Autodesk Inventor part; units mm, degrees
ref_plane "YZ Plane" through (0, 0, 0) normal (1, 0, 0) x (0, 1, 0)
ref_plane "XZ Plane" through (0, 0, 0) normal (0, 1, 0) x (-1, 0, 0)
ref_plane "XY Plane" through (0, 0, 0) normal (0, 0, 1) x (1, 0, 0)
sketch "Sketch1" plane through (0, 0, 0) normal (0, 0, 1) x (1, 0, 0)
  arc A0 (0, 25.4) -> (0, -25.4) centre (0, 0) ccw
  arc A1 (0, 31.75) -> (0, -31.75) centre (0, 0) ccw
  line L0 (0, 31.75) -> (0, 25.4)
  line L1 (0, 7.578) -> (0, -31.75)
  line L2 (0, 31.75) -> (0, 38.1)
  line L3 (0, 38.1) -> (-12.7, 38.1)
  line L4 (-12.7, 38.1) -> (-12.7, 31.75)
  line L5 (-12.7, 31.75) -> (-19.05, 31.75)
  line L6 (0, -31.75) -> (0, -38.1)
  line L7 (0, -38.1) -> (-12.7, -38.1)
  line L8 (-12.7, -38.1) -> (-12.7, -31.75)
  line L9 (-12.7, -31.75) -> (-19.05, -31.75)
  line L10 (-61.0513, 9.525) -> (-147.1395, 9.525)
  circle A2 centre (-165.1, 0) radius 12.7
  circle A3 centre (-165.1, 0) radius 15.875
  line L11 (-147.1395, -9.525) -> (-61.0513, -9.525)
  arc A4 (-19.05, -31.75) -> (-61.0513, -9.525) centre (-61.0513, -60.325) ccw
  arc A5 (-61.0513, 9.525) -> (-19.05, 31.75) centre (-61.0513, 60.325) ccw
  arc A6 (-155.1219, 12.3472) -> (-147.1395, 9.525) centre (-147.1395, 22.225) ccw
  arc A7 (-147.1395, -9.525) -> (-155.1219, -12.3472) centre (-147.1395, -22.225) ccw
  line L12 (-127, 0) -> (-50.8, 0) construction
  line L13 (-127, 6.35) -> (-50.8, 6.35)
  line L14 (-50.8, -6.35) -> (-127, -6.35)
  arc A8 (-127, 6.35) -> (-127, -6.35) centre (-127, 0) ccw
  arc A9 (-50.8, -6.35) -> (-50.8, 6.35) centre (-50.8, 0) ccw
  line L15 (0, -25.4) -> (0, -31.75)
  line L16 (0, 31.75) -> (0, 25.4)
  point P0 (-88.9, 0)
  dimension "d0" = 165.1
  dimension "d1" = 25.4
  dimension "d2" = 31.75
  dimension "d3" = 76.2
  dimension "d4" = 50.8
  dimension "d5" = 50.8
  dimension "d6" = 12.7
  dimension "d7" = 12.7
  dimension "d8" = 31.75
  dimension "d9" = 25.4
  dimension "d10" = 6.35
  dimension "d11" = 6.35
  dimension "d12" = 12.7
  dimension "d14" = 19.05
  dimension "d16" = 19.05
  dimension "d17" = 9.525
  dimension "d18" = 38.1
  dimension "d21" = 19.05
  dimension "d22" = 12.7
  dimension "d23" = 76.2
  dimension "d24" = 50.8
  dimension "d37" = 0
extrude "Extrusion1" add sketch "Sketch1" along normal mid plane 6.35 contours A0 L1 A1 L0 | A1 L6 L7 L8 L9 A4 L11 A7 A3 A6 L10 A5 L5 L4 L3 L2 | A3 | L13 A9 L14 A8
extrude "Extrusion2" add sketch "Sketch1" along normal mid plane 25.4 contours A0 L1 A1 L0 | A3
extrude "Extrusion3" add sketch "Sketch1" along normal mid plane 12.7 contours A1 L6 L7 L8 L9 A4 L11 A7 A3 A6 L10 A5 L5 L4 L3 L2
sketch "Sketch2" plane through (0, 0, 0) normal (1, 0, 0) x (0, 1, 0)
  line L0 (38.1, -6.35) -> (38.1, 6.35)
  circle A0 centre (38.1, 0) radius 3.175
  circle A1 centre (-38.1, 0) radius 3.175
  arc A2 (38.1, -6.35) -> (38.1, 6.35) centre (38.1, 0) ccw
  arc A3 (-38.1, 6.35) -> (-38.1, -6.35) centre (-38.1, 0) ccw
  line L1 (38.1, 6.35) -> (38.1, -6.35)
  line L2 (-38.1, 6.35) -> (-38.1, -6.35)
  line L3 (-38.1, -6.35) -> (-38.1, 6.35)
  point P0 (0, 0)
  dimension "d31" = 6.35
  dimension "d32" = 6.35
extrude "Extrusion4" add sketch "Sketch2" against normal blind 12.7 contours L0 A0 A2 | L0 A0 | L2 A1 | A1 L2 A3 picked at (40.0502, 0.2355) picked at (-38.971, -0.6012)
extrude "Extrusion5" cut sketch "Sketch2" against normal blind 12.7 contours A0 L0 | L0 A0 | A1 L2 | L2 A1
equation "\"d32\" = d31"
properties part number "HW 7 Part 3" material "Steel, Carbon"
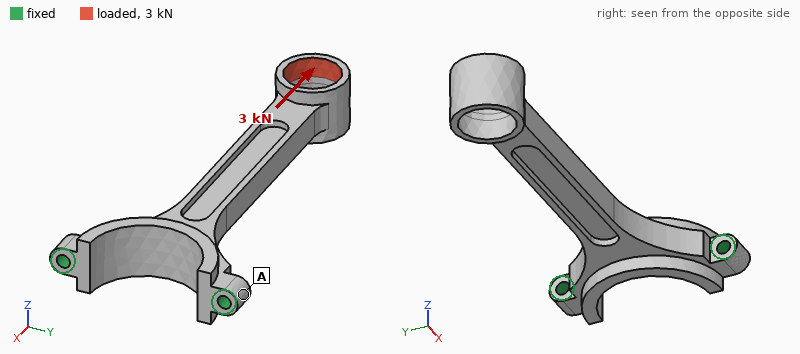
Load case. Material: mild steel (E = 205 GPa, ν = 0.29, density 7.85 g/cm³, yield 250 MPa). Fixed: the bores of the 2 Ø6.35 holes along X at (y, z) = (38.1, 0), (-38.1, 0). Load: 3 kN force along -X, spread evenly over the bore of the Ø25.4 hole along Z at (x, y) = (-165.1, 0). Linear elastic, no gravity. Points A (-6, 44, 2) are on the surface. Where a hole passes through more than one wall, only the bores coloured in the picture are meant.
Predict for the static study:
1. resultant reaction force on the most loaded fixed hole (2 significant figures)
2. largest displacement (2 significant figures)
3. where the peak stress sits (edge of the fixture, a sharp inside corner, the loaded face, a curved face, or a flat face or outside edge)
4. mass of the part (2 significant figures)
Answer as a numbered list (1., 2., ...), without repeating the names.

1. 1.9 kN
2. 0.90 mm
3. a curved face
4. 410 g
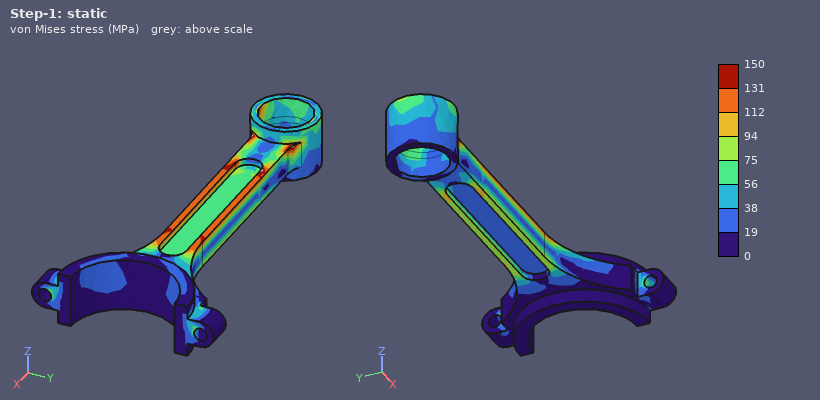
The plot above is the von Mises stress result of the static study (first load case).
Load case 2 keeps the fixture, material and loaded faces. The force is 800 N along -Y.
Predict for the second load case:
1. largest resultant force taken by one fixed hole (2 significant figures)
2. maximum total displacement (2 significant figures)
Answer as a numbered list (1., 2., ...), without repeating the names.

1. 2.4 kN
2. 0.60 mm
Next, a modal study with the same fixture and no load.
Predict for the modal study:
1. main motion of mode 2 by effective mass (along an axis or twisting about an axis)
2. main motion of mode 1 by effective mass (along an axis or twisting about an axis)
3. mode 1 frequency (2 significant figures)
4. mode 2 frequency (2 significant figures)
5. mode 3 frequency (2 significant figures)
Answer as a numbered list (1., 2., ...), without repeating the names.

1. along Y
2. along Z
3. 310 Hz
4. 710 Hz
5. 1800 Hz
